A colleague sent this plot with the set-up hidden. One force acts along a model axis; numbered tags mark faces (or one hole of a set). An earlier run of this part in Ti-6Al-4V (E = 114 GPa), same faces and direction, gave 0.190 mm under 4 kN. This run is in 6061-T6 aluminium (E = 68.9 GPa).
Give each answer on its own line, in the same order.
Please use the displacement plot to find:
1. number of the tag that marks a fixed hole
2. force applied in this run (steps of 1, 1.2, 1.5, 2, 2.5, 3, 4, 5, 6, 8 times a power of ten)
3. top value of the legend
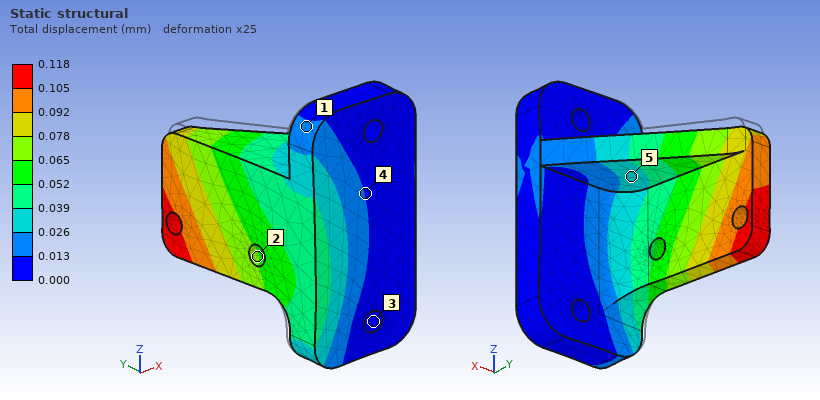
3
1.5 kN
0.118 mm
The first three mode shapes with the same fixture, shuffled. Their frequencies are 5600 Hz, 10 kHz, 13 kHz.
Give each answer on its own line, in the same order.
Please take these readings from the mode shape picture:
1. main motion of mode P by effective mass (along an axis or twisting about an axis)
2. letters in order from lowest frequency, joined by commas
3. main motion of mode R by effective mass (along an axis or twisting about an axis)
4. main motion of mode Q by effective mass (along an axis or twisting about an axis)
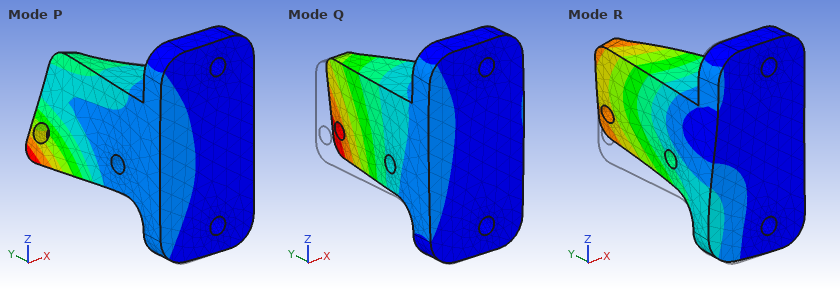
along Y
Q, R, P
along Z
along X
